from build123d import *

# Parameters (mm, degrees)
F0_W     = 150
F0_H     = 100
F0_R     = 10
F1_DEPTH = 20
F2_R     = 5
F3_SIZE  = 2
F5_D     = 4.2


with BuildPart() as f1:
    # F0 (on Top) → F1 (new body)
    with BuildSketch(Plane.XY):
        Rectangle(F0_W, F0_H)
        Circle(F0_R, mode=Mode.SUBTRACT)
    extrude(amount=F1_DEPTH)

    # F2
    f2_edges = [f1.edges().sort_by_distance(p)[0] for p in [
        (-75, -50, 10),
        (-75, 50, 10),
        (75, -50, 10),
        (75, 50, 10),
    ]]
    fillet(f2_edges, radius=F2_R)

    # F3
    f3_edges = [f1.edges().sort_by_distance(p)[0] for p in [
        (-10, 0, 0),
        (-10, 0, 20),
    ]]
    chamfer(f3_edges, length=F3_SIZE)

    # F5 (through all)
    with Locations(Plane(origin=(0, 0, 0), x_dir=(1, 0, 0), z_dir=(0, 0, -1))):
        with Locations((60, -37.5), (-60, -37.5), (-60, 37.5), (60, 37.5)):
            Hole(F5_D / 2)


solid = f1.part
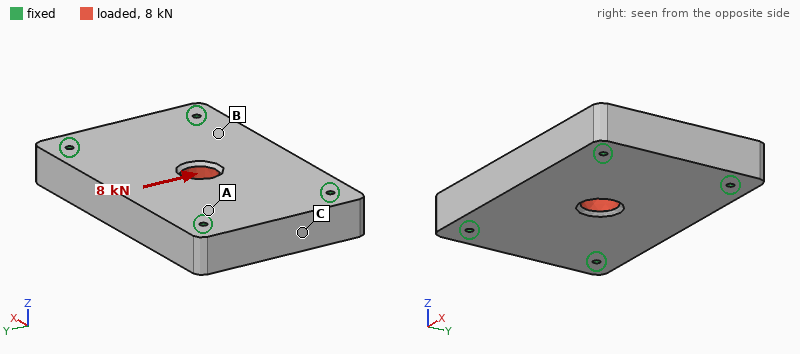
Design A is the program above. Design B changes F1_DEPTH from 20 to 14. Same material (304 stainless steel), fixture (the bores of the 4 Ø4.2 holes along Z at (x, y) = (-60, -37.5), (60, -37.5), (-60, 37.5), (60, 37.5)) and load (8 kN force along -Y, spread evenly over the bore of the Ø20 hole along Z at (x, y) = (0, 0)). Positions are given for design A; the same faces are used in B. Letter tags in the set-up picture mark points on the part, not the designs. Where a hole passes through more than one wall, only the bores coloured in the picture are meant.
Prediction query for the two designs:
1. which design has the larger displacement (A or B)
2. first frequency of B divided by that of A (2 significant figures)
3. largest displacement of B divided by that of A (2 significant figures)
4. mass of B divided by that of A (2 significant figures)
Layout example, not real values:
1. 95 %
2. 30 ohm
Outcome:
1. B
2. 0.77
3. 1.4
4. 0.70
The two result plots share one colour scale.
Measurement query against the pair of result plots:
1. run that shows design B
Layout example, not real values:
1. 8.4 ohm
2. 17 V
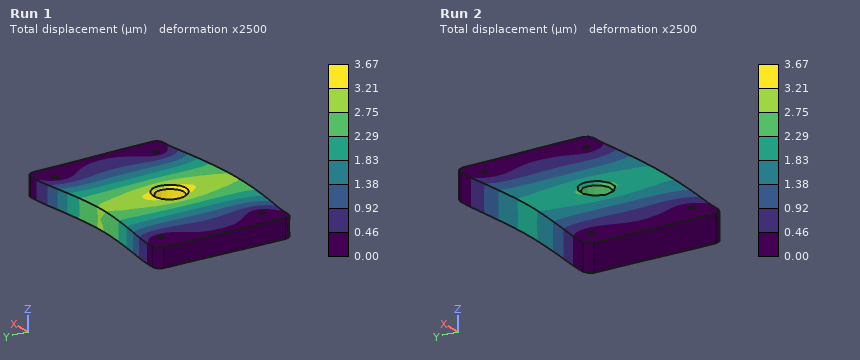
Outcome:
1. Run 1
